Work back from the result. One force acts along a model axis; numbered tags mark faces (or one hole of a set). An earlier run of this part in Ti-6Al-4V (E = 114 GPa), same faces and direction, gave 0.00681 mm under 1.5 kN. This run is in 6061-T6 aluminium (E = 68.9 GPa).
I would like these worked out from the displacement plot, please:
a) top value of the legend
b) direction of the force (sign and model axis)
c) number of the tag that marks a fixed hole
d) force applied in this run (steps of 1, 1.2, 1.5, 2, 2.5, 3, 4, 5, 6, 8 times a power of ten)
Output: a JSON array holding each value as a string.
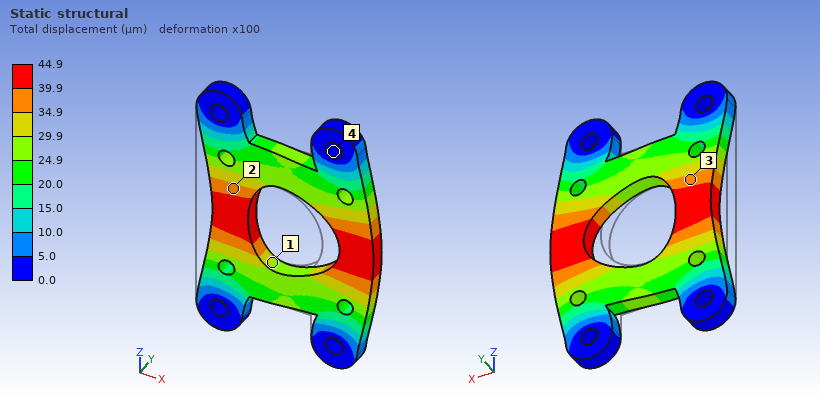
["44.9 µm", "+X", "4", "6 kN"]
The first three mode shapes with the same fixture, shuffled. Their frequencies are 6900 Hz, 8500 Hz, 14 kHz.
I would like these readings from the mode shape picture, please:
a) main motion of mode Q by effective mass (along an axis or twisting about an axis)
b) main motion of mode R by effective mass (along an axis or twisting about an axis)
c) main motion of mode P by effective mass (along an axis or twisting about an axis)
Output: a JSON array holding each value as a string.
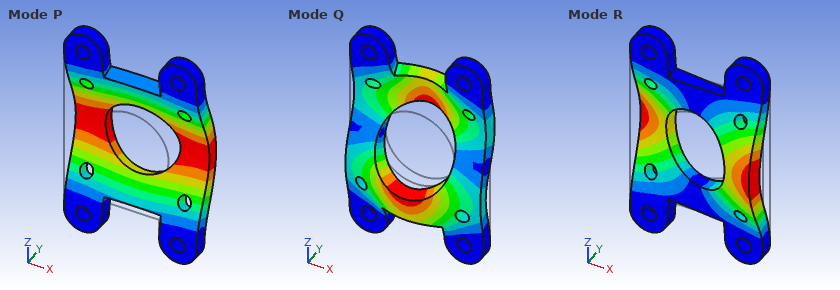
["twisting about X", "twisting about Z", "along Y"]
